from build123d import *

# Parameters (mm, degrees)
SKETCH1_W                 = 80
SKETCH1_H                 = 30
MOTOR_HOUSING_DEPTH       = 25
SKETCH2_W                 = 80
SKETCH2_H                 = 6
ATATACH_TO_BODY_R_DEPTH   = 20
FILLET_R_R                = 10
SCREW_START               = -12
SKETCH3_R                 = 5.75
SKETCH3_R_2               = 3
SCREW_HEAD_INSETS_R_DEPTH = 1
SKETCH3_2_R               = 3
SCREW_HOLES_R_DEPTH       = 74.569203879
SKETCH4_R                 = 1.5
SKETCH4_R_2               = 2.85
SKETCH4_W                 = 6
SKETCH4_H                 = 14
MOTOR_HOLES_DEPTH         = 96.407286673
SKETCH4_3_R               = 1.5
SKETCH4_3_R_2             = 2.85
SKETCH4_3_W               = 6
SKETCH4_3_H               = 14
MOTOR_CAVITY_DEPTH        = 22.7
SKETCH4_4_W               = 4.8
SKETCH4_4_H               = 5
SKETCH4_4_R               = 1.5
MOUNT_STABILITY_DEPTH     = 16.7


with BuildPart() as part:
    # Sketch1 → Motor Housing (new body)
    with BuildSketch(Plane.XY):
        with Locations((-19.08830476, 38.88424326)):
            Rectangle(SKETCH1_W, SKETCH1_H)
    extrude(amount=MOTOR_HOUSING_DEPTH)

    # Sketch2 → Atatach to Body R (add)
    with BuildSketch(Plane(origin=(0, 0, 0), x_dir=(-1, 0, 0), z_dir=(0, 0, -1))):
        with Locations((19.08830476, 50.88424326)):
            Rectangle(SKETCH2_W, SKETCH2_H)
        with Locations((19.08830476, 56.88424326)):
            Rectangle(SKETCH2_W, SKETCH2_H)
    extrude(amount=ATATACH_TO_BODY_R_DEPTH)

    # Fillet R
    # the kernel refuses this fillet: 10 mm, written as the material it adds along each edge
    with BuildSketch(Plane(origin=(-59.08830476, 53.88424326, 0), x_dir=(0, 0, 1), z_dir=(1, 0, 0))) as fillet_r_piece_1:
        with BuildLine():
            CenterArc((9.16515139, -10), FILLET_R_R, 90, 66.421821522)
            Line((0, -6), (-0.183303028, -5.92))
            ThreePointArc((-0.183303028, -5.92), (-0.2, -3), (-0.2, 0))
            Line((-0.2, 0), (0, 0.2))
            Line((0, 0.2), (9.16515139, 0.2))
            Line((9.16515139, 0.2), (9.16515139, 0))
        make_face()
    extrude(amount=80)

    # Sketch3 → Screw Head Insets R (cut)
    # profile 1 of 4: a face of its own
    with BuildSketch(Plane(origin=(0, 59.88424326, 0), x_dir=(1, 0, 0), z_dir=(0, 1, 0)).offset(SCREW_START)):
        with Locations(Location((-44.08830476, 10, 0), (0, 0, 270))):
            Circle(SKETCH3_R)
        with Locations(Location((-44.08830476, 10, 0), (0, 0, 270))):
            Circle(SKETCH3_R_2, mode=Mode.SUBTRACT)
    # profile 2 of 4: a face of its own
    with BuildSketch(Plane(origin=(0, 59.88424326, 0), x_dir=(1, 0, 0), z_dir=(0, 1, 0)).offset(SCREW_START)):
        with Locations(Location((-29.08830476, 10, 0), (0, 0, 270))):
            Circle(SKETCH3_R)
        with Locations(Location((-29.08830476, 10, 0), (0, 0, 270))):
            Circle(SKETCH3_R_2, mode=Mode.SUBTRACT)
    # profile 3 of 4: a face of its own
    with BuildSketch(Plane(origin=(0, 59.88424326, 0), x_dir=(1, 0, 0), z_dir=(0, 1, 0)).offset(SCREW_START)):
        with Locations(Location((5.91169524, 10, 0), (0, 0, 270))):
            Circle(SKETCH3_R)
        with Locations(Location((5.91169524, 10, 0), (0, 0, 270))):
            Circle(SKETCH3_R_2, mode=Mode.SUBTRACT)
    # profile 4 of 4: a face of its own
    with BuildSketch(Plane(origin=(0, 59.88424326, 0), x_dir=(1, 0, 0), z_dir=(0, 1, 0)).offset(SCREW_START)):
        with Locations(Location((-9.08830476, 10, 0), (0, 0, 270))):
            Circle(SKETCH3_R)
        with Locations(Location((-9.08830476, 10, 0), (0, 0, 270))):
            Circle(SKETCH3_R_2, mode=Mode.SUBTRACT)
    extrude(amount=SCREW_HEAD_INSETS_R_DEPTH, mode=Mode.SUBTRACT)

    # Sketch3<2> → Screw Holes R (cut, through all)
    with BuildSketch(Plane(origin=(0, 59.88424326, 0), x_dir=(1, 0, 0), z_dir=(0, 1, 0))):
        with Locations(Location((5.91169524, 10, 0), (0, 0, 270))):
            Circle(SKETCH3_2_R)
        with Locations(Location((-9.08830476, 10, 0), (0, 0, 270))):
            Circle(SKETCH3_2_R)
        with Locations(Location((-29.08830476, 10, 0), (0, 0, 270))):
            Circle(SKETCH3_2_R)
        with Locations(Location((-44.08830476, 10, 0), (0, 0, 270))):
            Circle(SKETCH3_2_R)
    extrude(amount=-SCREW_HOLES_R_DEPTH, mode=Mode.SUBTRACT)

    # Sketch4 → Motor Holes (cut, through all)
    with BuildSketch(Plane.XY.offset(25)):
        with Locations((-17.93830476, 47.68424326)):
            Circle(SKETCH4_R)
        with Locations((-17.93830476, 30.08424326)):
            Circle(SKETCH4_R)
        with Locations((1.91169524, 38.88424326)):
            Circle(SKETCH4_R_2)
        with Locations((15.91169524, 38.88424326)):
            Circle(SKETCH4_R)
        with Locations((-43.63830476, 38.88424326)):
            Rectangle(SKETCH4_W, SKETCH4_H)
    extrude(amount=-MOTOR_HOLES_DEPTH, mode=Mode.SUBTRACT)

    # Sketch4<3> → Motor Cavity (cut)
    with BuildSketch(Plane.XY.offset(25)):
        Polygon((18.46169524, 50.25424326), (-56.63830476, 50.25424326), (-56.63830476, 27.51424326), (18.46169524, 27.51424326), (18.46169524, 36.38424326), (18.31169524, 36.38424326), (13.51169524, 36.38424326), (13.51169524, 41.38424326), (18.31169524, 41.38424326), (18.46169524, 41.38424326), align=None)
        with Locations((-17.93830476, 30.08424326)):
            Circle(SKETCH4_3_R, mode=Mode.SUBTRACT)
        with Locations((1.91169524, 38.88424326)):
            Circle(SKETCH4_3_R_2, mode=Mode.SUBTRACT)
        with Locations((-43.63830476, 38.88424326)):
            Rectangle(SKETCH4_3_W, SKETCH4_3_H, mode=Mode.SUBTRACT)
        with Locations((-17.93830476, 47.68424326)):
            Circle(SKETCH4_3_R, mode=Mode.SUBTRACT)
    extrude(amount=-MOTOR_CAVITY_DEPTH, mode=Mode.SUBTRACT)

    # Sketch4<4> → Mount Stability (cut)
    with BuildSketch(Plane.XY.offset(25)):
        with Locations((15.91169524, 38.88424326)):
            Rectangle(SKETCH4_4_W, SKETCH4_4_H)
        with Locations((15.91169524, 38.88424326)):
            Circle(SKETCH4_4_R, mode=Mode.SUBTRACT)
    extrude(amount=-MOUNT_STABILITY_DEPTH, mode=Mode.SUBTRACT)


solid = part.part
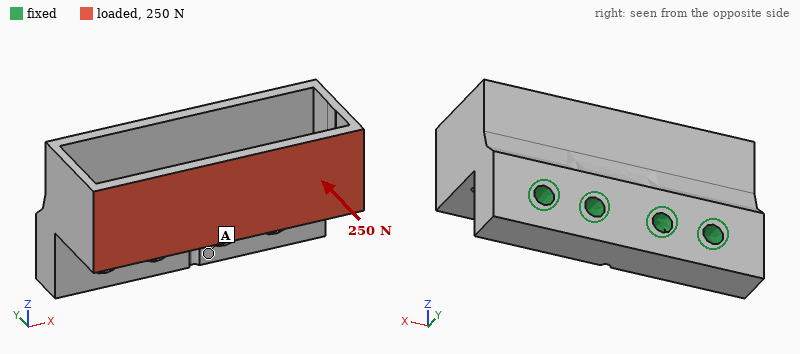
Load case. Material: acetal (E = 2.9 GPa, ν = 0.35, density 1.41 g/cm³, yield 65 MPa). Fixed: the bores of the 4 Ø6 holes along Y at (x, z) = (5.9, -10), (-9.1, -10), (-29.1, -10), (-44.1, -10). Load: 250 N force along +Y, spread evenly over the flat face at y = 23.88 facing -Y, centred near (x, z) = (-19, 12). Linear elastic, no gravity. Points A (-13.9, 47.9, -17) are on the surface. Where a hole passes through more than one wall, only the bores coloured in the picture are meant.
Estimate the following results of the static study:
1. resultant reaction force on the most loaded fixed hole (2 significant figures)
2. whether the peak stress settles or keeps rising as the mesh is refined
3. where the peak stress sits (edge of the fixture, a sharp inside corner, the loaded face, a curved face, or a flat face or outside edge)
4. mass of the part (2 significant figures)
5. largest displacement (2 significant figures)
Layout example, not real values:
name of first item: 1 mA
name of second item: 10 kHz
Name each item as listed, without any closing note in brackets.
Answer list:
resultant reaction force on the most loaded fixed hole: 69 N
whether the peak stress settles or keeps rising as the mesh is refined: keeps rising
where the peak stress sits: a sharp inside corner
mass of the part: 56 g
largest displacement: 1.2 mm
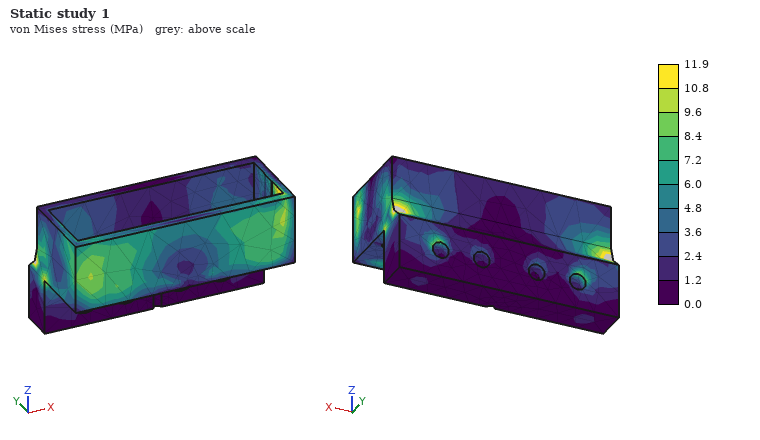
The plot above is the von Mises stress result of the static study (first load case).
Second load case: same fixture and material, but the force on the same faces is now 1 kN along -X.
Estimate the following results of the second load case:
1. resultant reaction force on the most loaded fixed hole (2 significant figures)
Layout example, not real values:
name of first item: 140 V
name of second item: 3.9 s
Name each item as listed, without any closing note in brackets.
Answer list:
resultant reaction force on the most loaded fixed hole: 670 N
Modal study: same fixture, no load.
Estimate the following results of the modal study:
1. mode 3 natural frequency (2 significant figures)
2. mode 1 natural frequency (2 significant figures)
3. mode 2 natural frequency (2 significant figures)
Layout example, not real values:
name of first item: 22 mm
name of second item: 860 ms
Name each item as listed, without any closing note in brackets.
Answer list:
mode 3 natural frequency: 1400 Hz
mode 1 natural frequency: 690 Hz
mode 2 natural frequency: 1000 Hz
